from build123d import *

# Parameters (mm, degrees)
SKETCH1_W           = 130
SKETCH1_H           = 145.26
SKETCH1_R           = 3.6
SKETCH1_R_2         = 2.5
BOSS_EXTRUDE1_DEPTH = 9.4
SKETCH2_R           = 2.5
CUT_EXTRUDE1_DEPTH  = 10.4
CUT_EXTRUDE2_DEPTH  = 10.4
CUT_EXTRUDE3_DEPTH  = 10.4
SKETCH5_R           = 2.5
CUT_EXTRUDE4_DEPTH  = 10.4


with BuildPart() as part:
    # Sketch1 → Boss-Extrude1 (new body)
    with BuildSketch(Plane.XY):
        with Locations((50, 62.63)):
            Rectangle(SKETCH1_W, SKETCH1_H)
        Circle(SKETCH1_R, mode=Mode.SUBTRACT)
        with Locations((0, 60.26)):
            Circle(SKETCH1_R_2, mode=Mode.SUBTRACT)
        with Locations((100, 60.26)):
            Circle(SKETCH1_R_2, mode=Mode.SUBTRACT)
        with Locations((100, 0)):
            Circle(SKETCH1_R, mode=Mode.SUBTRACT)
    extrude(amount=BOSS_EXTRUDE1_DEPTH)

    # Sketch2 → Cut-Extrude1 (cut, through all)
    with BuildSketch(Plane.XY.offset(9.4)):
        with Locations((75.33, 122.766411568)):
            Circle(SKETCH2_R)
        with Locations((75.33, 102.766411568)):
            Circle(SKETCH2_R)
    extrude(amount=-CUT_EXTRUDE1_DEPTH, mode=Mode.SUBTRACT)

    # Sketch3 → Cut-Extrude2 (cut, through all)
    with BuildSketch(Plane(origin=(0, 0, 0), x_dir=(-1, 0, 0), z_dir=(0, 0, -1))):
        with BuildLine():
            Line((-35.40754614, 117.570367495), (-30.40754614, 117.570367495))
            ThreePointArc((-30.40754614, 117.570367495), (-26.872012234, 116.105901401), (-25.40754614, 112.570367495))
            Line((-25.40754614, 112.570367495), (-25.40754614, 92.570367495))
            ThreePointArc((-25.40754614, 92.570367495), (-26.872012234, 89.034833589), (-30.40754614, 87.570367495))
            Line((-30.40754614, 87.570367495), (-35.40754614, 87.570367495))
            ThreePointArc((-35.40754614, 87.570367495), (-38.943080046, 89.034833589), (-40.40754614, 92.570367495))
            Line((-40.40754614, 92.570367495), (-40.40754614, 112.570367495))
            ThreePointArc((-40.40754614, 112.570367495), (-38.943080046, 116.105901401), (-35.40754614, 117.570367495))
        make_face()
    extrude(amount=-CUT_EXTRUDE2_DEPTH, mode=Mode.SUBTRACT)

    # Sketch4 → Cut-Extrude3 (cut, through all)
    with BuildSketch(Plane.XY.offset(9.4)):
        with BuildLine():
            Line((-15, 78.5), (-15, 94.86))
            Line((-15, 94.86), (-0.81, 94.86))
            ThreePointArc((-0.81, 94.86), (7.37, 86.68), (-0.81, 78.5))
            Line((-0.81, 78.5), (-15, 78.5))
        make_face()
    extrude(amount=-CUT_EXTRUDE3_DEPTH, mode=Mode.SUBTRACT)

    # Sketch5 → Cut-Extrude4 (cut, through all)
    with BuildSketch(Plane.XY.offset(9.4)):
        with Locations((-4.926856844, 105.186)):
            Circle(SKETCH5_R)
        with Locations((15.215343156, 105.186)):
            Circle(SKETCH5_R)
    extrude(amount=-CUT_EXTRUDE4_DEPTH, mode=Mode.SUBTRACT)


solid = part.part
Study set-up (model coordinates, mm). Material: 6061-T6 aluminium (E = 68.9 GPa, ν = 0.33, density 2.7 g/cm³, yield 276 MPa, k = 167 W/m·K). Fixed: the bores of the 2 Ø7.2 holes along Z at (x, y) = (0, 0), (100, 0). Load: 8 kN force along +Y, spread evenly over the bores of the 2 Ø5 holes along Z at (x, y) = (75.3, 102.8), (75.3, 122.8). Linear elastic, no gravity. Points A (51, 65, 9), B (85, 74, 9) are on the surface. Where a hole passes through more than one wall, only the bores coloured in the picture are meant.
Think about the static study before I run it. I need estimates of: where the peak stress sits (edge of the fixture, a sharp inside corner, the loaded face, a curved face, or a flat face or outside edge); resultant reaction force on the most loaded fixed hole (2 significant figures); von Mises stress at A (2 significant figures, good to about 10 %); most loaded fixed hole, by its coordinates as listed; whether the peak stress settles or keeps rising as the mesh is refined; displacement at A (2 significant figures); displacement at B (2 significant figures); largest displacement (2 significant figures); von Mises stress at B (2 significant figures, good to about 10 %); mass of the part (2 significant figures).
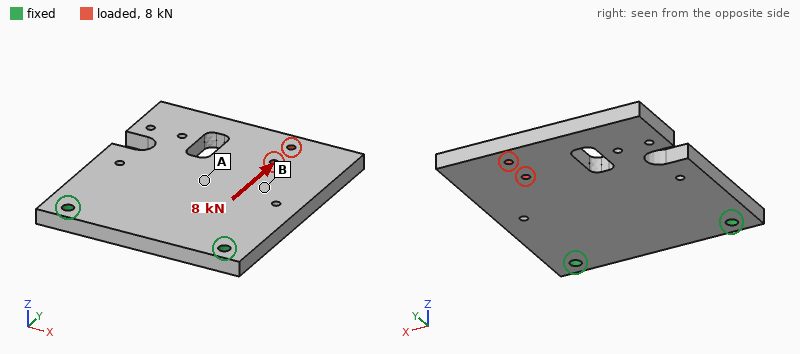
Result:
edge of the fixture
6.1 kN
7.4 MPa
(100, 0)
keeps rising
13 µm
19 µm
32 µm
14 MPa
450 g
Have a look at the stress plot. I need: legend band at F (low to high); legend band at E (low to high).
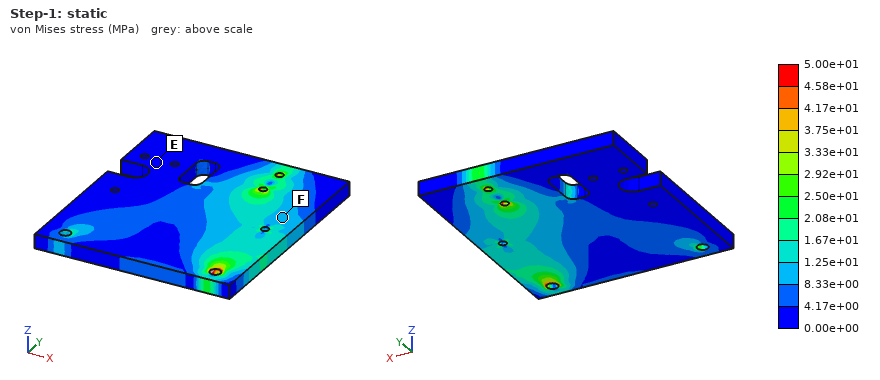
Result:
8.33e+00 to 1.25e+01 MPa
0.00e+00 to 4.17e+00 MPa
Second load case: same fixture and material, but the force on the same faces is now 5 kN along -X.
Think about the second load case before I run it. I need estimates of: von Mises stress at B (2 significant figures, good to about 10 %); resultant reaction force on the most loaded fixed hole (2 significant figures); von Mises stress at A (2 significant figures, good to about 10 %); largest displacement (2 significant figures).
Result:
10 MPa
6.1 kN
9.8 MPa
70 µm
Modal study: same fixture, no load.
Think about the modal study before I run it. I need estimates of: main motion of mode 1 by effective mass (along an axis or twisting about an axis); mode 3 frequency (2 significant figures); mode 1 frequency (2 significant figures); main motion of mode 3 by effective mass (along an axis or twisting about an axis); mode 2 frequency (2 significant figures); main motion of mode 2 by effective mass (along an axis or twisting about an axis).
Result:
along Z
2200 Hz
370 Hz
along Z
1000 Hz
twisting about Y
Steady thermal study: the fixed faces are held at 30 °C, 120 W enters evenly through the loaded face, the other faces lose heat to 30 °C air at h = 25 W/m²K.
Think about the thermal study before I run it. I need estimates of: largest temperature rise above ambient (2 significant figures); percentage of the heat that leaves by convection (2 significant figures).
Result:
87 K
31 %
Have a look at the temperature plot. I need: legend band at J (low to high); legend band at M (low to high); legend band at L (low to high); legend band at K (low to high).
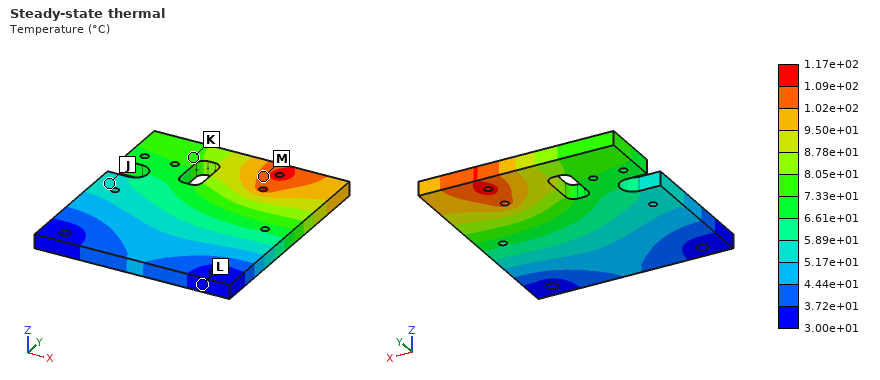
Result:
5.17e+01 to 5.89e+01 °C
1.02e+02 to 1.09e+02 °C
3.00e+01 to 3.72e+01 °C
7.33e+01 to 8.05e+01 °C
